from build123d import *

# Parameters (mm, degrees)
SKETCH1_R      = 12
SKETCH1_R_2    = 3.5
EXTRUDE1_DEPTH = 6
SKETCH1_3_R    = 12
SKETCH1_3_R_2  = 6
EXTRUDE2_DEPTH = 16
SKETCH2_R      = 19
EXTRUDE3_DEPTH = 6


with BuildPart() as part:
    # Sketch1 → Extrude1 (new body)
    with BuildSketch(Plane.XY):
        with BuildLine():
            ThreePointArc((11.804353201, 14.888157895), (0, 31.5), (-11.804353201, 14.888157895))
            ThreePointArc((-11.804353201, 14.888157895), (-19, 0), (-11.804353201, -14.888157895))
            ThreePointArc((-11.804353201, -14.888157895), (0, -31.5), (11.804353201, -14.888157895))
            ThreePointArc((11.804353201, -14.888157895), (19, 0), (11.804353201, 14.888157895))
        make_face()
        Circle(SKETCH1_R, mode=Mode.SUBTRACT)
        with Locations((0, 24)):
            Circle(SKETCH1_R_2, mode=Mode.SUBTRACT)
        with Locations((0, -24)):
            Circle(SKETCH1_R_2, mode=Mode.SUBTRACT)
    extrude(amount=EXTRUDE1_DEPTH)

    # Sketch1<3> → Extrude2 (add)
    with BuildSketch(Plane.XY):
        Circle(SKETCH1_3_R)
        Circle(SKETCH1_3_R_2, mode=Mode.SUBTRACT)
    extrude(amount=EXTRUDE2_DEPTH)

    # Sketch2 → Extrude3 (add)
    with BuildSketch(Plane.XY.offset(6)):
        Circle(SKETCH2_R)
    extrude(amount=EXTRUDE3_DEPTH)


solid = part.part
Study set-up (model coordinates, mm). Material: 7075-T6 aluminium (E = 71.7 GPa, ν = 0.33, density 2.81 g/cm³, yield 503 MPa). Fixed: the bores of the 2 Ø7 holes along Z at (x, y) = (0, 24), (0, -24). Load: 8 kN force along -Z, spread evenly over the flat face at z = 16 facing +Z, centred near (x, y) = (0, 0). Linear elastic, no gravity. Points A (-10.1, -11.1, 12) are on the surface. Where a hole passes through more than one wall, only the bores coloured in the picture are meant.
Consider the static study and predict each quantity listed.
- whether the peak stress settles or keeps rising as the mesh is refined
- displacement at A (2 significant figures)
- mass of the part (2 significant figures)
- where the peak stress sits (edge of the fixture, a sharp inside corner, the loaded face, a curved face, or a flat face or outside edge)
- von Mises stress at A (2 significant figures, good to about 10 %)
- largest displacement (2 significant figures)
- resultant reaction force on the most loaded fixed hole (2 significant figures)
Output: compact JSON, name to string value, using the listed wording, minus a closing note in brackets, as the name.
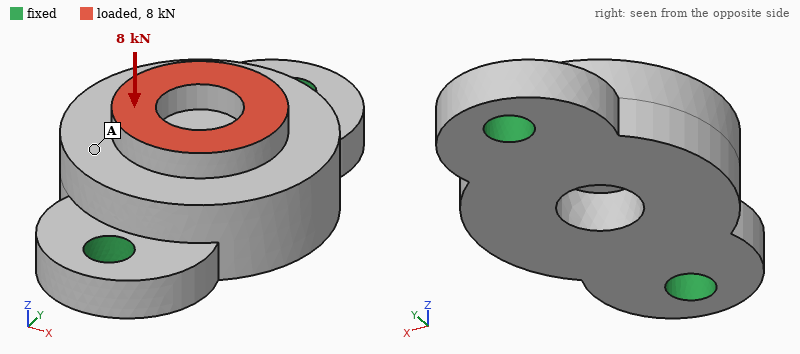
{"whether the peak stress settles or keeps rising as the mesh is refined": "keeps rising", "displacement at A": "25 µm", "mass of the part": "48 g", "where the peak stress sits": "edge of the fixture", "von Mises stress at A": "34 MPa", "largest displacement": "34 µm", "resultant reaction force on the most loaded fixed hole": "5.1 kN"}
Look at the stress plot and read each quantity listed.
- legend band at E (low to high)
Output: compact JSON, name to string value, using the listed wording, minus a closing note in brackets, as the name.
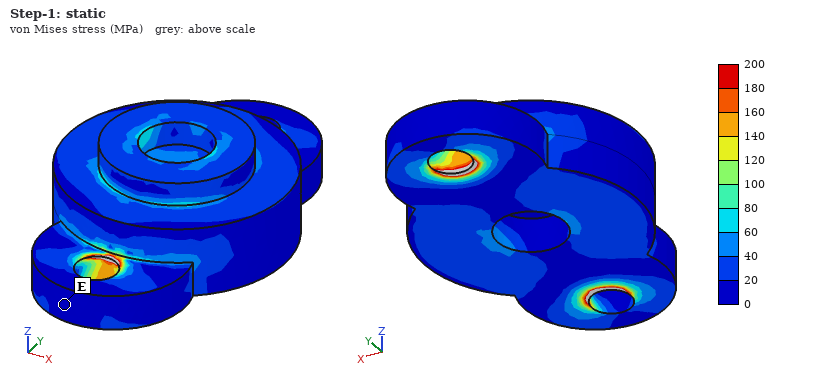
{"legend band at E": "0 to 20 MPa"}
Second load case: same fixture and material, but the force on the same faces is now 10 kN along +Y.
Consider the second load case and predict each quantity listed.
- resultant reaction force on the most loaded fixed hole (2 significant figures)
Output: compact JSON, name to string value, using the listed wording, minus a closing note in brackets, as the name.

{"resultant reaction force on the most loaded fixed hole": "5.9 kN"}
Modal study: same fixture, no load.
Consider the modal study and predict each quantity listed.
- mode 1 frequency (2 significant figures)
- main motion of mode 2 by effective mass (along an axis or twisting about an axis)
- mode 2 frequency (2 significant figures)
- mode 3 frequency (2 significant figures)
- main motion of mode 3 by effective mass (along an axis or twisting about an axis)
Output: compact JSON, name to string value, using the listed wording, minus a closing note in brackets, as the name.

{"mode 1 frequency": "8400 Hz", "main motion of mode 2 by effective mass": "along Z", "mode 2 frequency": "14 kHz", "mode 3 frequency": "21 kHz", "main motion of mode 3 by effective mass": "along X"}
